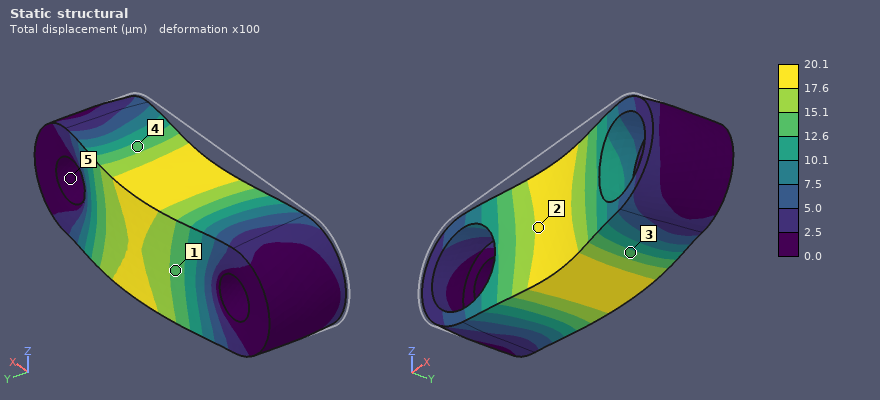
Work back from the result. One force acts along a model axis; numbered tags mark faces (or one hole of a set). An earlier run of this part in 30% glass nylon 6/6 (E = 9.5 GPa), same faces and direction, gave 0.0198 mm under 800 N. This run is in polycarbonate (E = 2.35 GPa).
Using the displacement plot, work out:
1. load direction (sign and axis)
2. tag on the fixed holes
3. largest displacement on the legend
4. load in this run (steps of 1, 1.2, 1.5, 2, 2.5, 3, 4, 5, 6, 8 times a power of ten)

+Y
5
20.1 µm
200 N
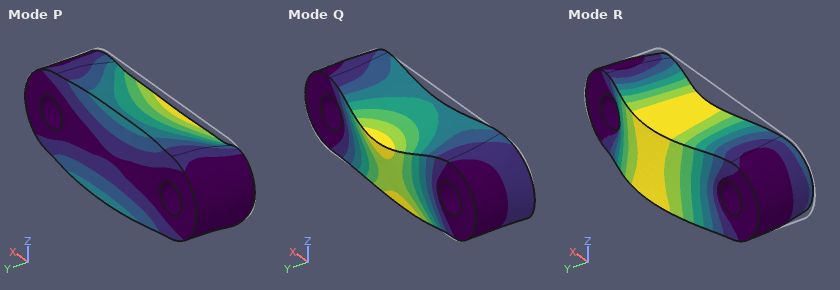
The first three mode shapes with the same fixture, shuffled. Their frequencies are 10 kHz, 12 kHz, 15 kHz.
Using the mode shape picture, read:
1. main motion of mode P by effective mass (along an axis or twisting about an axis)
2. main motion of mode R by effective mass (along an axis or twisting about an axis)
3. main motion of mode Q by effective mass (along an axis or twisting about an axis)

along Z
along Y
along Z
